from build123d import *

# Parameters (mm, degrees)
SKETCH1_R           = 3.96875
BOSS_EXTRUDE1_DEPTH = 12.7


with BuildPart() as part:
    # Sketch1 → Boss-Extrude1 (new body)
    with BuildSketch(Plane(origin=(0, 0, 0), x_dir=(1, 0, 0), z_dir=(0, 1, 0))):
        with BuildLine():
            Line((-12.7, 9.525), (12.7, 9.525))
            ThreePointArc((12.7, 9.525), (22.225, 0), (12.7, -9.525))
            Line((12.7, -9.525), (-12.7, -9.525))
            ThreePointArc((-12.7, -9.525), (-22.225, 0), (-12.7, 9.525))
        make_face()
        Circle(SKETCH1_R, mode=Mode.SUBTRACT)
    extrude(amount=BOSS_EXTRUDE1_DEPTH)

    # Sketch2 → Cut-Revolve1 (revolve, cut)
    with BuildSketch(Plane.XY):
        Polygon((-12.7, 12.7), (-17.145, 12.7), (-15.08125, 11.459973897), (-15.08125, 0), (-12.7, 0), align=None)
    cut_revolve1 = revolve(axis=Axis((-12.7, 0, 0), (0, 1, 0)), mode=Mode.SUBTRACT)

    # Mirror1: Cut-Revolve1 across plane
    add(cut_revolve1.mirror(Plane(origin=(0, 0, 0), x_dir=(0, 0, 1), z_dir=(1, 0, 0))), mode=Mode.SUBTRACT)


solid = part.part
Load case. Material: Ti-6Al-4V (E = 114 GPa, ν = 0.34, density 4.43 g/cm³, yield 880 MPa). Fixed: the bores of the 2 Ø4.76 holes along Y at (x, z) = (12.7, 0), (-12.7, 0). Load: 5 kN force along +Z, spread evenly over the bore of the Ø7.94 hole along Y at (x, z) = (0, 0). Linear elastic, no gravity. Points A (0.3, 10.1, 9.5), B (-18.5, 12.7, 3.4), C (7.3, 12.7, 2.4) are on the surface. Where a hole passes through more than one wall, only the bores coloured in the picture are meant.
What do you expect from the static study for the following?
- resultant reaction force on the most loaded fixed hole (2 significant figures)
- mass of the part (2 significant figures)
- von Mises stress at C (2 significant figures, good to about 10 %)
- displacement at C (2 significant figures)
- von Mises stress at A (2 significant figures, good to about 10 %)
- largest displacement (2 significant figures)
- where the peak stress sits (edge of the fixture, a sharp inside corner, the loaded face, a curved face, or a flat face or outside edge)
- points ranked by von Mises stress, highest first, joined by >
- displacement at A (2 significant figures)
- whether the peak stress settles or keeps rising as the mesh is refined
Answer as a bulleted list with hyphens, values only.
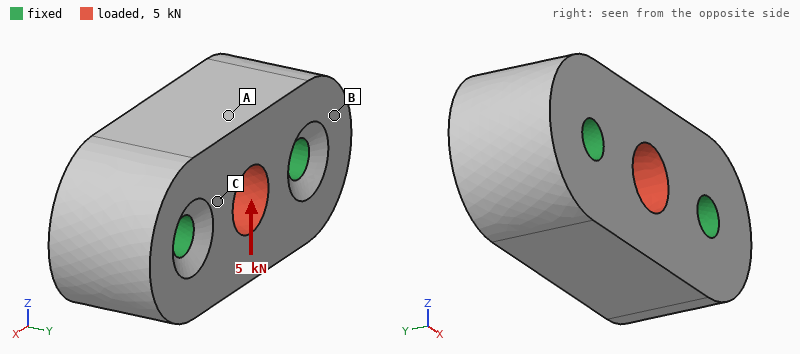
- 2.5 kN
- 38 g
- 22 MPa
- 2.1 µm
- 34 MPa
- 4.5 µm
- edge of the fixture
- A > C > B
- 3.6 µm
- keeps rising
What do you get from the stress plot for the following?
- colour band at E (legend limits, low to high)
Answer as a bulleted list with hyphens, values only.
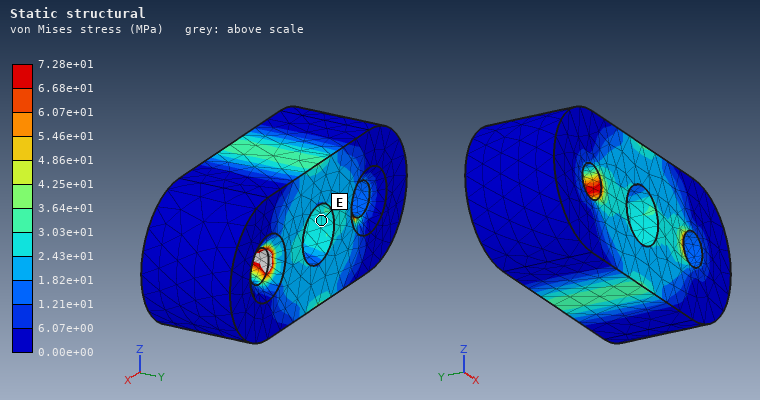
- 2.43e+01 to 3.03e+01 MPa
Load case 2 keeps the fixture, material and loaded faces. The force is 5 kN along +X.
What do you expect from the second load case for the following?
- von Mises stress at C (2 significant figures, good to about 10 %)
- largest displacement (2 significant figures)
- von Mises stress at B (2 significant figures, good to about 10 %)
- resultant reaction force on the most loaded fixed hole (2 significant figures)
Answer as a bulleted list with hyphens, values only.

- 15 MPa
- 1.7 µm
- 3.8 MPa
- 2.5 kN
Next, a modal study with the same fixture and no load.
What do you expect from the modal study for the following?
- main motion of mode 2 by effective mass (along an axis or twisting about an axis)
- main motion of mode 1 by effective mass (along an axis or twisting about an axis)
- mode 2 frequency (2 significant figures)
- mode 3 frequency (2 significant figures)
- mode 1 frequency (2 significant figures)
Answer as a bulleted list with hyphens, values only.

- along Y
- twisting about X
- 47 kHz
- 51 kHz
- 45 kHz
